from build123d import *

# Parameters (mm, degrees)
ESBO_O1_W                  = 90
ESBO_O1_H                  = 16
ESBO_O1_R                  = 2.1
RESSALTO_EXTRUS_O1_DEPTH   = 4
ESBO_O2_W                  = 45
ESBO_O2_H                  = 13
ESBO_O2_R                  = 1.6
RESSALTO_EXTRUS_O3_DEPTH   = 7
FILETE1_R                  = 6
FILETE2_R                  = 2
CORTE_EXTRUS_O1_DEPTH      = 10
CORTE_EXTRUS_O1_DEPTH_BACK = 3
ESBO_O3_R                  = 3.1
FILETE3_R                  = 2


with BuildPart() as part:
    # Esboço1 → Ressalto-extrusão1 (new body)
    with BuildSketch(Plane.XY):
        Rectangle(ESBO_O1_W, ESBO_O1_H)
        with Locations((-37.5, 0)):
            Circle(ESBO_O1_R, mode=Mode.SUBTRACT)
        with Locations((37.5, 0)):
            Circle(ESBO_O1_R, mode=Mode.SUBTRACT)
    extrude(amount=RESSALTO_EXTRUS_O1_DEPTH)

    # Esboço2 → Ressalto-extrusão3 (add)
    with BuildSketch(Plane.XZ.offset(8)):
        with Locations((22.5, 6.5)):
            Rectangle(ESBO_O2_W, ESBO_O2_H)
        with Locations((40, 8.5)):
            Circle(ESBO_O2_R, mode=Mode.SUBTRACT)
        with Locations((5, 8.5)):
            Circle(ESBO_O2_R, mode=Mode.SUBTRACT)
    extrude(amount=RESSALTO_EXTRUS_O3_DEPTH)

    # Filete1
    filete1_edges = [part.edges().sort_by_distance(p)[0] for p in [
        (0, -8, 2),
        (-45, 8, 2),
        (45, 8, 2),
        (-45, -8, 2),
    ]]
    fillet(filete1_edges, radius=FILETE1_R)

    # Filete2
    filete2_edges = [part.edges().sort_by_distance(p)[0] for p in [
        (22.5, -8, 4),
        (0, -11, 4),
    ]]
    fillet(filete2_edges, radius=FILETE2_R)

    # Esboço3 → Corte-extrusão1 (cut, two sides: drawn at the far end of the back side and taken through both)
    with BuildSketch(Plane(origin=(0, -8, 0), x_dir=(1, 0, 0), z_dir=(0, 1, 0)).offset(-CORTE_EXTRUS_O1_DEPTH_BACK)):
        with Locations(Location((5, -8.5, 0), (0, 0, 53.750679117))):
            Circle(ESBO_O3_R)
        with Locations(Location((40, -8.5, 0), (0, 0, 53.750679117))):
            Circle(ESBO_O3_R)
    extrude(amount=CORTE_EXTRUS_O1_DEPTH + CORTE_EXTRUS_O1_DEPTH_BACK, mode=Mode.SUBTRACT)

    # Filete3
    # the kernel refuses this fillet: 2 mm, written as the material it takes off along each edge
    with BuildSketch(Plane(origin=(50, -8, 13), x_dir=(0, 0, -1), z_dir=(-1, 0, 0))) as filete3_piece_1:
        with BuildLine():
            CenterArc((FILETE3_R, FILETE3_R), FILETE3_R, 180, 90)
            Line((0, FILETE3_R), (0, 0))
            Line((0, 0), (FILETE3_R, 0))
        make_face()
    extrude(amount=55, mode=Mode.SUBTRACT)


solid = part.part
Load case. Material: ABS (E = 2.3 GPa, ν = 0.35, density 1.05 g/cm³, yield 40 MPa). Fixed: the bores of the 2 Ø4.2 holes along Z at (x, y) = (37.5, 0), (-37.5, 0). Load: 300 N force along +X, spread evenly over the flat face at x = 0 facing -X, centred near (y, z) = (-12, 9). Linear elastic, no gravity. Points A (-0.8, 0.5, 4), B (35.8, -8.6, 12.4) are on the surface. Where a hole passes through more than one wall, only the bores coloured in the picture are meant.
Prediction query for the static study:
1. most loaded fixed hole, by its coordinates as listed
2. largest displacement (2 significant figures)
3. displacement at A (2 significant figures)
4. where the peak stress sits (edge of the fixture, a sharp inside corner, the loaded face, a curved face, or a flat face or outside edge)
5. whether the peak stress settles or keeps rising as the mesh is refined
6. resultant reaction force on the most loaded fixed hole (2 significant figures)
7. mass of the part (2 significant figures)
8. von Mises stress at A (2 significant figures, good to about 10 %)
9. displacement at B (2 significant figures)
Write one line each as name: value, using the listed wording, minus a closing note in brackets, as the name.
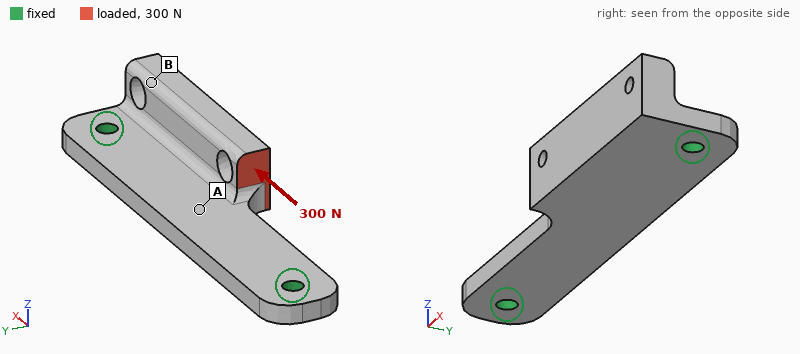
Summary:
most loaded fixed hole, by its coordinates as listed: (37.5, 0)
largest displacement: 0.65 mm
displacement at A: 0.40 mm
where the peak stress sits: edge of the fixture
whether the peak stress settles or keeps rising as the mesh is refined: keeps rising
resultant reaction force on the most loaded fixed hole: 210 N
mass of the part: 9.9 g
von Mises stress at A: 7.1 MPa
displacement at B: 0.19 mm
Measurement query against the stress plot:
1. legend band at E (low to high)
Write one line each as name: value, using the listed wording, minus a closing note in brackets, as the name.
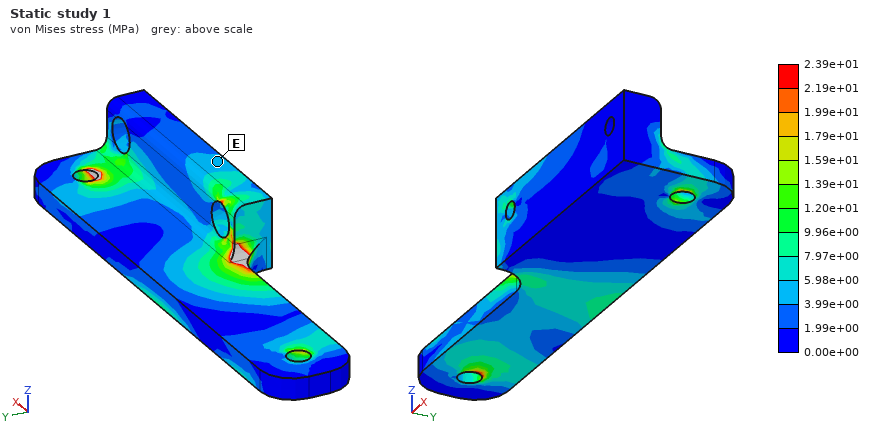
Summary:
legend band at E: 3.99e+00 to 5.98e+00 MPa
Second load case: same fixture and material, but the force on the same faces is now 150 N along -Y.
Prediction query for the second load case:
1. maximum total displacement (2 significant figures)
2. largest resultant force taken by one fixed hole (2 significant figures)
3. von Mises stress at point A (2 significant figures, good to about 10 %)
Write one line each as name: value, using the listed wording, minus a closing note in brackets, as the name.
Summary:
maximum total displacement: 0.95 mm
largest resultant force taken by one fixed hole: 79 N
von Mises stress at point A: 4.4 MPa
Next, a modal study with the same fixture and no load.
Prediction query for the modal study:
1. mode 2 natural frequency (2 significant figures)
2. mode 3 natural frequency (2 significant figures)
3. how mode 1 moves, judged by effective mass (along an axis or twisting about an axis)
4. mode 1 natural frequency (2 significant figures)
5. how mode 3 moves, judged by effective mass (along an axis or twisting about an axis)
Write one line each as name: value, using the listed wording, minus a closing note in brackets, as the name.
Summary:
mode 2 natural frequency: 1500 Hz
mode 3 natural frequency: 2300 Hz
how mode 1 moves, judged by effective mass: along Z
mode 1 natural frequency: 920 Hz
how mode 3 moves, judged by effective mass: along Y
